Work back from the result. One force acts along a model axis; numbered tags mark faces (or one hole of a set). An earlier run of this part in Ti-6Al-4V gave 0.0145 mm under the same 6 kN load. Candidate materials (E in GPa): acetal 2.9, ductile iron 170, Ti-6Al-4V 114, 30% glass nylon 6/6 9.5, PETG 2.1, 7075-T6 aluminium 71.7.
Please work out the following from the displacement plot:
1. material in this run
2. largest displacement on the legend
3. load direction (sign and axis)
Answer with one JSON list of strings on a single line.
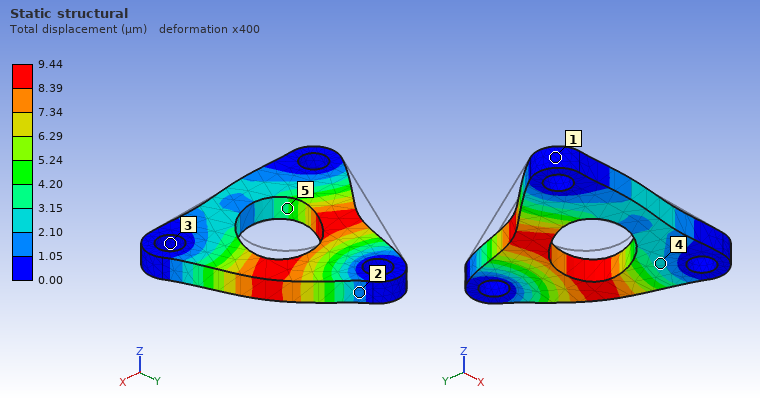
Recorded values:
["ductile iron", "9.44 µm", "+X"]
